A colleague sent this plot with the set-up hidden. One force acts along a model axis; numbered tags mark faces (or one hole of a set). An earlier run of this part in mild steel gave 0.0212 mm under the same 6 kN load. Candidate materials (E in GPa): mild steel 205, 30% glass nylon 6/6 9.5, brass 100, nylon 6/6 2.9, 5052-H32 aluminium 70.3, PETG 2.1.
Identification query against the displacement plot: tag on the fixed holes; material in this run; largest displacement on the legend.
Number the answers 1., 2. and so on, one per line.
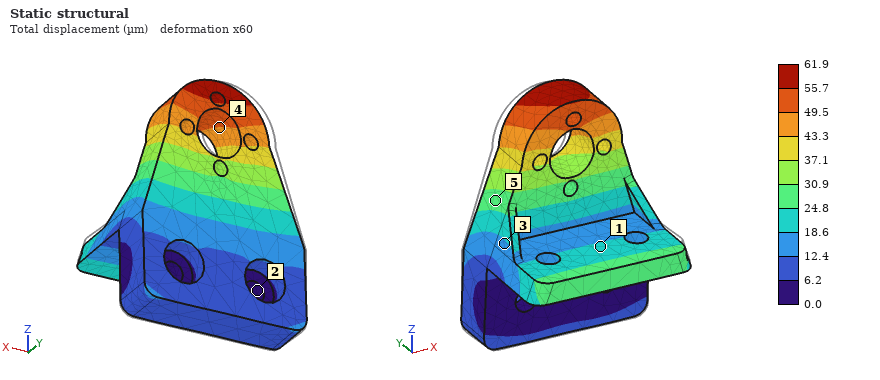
1. 2
2. 5052-H32 aluminium
3. 61.9 µm
